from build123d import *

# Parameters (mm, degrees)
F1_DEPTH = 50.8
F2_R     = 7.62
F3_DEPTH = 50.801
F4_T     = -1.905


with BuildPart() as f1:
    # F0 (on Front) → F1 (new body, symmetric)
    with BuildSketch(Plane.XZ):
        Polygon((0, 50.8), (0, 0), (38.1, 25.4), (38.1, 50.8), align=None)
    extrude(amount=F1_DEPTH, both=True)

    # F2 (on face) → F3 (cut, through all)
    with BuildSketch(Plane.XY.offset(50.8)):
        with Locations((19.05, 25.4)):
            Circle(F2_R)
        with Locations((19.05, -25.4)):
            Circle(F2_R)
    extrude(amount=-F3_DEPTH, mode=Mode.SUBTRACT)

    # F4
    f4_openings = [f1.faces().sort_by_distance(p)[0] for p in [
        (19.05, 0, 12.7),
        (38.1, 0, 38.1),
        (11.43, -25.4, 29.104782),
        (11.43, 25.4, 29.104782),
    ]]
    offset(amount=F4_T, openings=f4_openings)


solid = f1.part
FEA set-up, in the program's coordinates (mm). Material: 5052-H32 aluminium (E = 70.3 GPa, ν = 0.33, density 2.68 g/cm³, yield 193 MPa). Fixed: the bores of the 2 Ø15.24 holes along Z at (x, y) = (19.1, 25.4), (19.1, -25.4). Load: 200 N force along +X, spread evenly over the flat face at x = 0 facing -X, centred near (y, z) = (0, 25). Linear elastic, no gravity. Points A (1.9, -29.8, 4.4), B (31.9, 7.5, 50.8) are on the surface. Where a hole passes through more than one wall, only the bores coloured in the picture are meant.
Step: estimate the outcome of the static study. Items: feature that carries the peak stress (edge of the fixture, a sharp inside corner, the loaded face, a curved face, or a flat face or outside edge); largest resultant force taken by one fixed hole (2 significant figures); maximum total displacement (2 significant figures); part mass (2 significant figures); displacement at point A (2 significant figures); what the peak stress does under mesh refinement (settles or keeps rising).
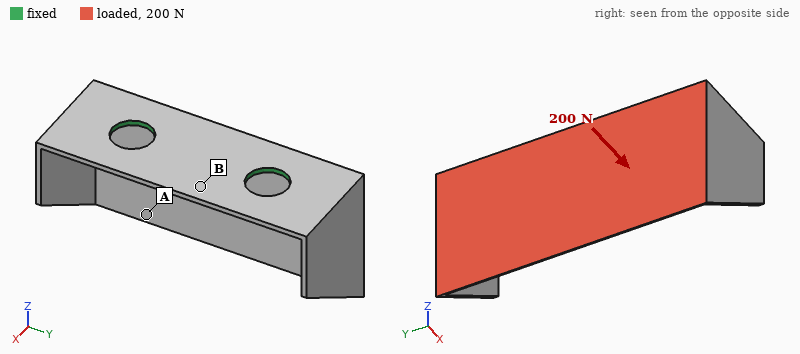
edge of the fixture
100 N
0.60 mm
56 g
0.42 mm
keeps rising
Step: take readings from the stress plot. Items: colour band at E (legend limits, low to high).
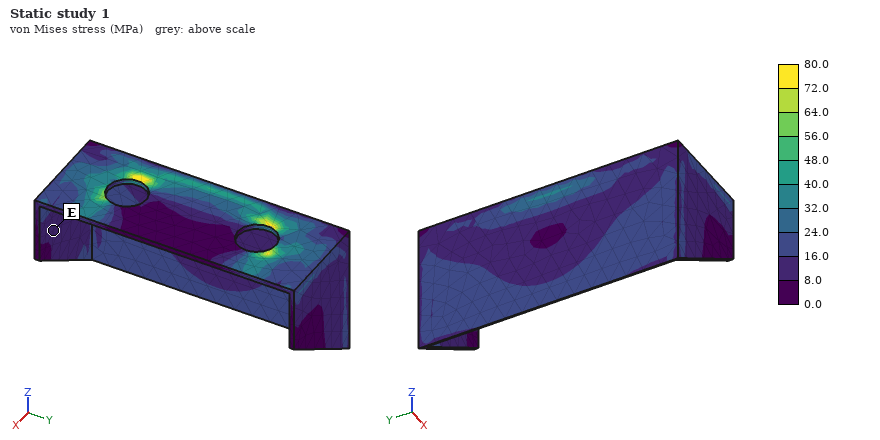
8.0 to 16.0 MPa
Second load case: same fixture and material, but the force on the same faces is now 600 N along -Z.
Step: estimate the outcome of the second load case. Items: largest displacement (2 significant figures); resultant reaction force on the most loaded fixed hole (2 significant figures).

0.44 mm
300 N
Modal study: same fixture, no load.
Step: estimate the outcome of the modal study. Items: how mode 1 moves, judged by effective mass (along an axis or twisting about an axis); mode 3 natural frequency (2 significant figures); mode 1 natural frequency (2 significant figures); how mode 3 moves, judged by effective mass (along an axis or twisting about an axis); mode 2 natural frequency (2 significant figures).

along X
1700 Hz
710 Hz
along Y
1000 Hz
